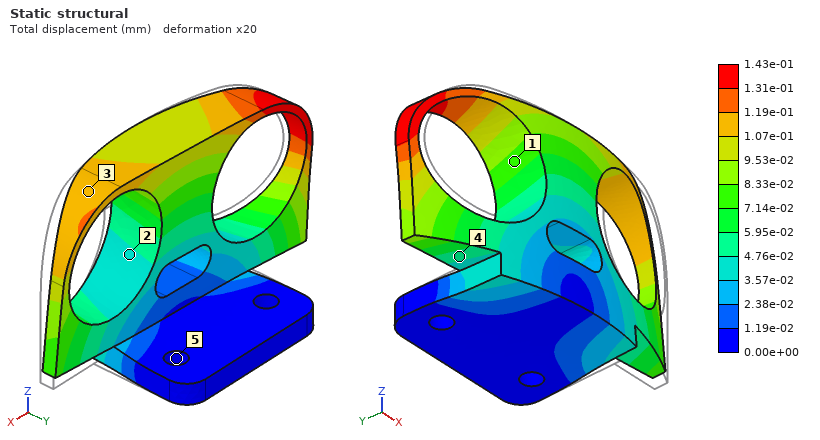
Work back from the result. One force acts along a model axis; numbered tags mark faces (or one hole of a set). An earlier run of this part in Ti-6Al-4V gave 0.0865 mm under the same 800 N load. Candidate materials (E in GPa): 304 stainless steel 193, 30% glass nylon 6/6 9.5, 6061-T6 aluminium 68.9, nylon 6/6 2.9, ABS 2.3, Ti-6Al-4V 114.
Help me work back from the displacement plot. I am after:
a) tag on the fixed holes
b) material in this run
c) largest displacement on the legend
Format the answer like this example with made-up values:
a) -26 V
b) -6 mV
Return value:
a) 5
b) 6061-T6 aluminium
c) 1.43e-01 mm
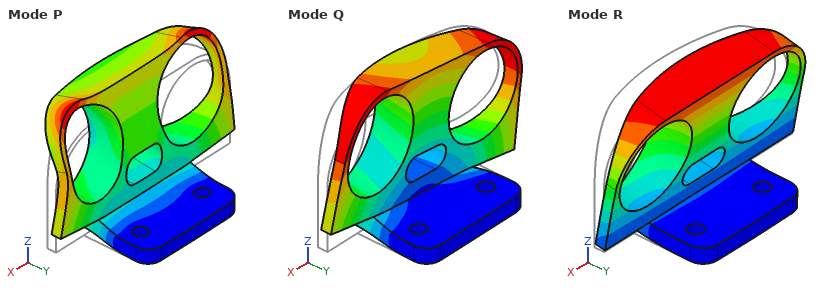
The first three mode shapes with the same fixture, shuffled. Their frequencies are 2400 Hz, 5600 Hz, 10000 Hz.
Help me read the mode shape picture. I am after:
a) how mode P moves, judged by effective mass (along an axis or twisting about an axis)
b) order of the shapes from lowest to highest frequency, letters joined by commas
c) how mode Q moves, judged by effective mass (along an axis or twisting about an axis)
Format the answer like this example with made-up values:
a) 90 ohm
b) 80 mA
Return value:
a) along Z
b) R, Q, P
c) along X
